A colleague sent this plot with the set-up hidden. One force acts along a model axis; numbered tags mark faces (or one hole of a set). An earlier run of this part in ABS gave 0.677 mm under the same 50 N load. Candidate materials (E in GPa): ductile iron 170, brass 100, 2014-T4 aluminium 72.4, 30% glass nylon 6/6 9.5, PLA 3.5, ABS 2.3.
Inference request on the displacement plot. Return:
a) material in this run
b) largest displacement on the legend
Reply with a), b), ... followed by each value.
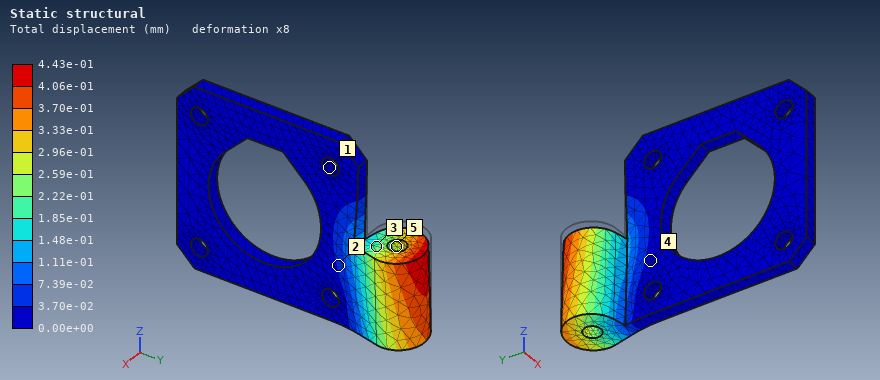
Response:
a) PLA
b) 4.43e-01 mm
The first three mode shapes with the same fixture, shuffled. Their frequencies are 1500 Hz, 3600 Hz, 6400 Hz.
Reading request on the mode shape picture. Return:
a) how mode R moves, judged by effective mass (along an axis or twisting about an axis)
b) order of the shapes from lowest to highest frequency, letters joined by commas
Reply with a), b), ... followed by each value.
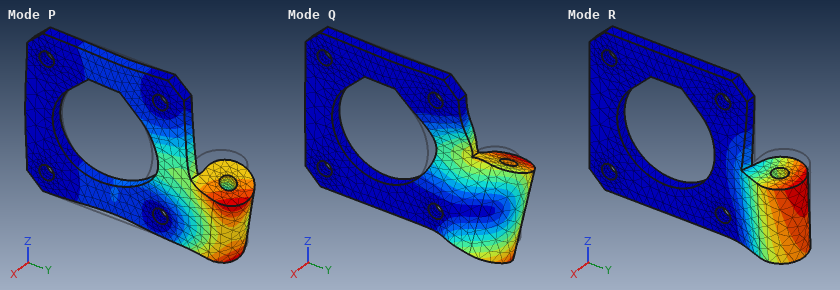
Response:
a) along X
b) R, Q, P
